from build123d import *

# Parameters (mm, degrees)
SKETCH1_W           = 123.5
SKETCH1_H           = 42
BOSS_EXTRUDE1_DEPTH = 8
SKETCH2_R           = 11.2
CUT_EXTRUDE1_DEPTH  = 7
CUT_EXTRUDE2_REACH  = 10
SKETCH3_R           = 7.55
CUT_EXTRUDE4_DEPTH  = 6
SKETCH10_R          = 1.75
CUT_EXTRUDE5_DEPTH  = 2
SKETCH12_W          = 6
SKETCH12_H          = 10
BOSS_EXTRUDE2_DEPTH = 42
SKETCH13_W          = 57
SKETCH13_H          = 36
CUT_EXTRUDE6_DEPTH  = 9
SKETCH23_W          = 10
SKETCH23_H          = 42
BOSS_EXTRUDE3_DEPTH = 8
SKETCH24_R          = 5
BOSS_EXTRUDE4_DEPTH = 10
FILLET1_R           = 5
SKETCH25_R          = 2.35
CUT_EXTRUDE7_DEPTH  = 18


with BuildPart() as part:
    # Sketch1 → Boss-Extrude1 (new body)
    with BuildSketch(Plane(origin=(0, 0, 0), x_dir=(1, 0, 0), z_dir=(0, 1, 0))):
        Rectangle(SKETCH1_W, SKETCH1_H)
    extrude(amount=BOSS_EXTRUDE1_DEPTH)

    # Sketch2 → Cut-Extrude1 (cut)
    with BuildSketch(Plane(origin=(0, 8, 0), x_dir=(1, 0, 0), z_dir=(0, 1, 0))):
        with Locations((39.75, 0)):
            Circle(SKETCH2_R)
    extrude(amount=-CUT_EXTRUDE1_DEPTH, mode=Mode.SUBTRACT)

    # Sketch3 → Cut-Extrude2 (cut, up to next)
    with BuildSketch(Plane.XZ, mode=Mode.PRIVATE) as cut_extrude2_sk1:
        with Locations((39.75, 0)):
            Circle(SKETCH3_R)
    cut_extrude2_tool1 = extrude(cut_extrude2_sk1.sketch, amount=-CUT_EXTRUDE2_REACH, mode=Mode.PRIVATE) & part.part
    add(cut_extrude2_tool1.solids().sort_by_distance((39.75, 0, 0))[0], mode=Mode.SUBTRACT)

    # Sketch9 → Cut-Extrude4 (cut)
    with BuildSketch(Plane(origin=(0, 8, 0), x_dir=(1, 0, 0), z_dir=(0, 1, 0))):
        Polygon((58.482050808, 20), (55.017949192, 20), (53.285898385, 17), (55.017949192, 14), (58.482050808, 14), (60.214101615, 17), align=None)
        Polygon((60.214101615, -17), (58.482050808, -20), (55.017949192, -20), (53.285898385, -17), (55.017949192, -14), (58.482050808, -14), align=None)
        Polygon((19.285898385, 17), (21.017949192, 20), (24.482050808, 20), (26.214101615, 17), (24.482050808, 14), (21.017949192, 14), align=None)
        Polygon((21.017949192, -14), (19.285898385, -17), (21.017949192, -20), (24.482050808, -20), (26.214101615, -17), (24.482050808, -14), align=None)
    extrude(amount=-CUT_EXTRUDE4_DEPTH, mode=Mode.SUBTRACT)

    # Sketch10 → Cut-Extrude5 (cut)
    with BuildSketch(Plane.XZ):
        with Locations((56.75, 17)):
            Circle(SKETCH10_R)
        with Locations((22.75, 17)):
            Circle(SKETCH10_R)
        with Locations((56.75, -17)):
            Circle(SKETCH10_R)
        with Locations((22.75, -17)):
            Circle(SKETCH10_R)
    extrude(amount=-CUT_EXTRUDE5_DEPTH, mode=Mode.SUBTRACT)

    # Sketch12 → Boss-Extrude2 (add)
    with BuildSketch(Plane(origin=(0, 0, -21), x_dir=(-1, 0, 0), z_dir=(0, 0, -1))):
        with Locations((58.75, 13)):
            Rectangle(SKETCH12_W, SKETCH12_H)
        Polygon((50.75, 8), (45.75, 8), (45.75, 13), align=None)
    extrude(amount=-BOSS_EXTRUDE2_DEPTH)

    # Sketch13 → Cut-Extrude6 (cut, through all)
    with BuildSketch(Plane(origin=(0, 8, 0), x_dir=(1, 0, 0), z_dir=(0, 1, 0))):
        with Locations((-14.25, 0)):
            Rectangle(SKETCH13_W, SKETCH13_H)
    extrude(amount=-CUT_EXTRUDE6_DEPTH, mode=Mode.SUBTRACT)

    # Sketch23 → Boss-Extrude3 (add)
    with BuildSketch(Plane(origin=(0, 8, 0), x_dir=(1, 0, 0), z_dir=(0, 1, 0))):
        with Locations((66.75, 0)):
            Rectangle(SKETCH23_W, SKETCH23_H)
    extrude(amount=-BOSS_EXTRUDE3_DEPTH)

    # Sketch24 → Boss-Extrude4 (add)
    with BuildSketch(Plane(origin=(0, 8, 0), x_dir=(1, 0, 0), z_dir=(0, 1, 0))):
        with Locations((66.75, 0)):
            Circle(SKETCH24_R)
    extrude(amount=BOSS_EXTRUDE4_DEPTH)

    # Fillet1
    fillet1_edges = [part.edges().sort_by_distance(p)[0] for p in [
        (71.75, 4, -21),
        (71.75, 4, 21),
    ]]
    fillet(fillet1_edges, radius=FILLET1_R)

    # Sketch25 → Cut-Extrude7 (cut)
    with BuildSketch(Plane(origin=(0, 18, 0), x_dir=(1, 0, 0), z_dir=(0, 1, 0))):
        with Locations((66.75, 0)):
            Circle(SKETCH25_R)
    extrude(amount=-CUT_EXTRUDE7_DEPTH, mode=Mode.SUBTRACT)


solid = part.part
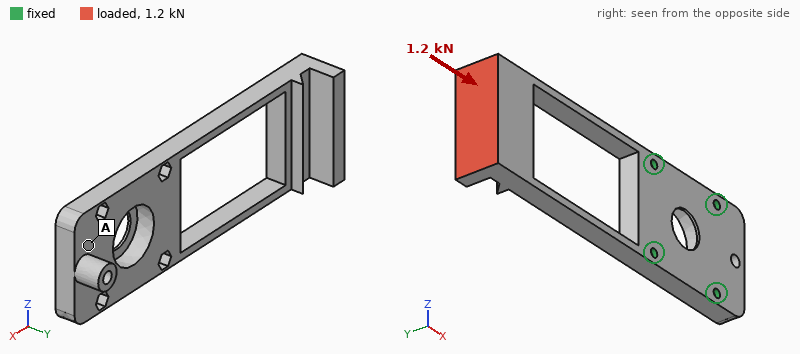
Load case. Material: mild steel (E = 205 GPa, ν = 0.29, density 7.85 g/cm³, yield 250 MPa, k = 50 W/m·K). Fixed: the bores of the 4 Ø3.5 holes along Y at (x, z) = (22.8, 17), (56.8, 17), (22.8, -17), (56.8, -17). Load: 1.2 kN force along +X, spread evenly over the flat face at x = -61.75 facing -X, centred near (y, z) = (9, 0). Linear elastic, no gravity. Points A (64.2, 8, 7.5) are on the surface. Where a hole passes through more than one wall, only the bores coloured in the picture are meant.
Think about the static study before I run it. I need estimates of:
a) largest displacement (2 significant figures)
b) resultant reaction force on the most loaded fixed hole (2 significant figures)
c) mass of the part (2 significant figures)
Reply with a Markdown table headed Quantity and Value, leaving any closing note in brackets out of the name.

| Quantity | Value |
|---|---|
| largest displacement | 0.42 mm |
| resultant reaction force on the most loaded fixed hole | 390 N |
| mass of the part | 220 g |
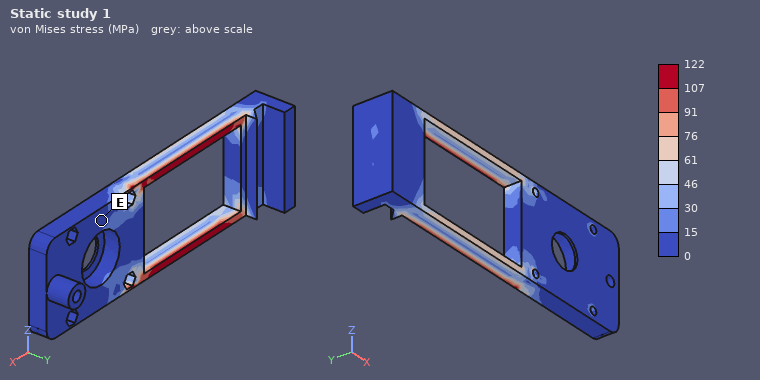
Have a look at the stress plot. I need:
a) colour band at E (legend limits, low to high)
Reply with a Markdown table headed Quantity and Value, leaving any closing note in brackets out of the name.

| Quantity | Value |
|---|---|
| colour band at E | 0 to 15 MPa |
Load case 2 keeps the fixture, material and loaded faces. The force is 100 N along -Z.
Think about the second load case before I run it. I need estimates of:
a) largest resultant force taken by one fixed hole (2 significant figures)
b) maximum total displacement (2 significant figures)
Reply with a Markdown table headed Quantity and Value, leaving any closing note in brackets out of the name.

| Quantity | Value |
|---|---|
| largest resultant force taken by one fixed hole | 200 N |
| maximum total displacement | 0.26 mm |
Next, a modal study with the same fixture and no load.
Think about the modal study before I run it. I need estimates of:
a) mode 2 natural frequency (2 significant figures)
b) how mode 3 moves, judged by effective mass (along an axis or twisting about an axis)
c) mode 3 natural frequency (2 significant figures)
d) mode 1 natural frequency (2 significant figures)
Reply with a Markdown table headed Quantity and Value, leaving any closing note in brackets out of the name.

| Quantity | Value |
|---|---|
| mode 2 natural frequency | 350 Hz |
| how mode 3 moves, judged by effective mass | twisting about X |
| mode 3 natural frequency | 1200 Hz |
| mode 1 natural frequency | 340 Hz |
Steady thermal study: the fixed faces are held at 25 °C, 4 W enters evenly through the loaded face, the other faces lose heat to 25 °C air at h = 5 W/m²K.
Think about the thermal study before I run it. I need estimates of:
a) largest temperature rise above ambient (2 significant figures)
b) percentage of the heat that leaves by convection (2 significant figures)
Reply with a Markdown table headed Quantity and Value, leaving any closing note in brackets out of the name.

| Quantity | Value |
|---|---|
| largest temperature rise above ambient | 75 K |
| percentage of the heat that leaves by convection | 40 % |
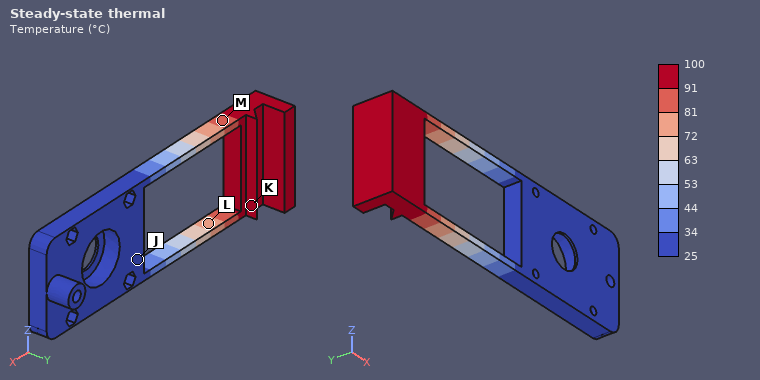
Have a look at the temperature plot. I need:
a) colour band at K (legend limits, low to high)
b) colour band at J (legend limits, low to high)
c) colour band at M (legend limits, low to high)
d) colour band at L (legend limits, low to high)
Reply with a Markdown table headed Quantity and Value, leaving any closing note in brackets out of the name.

| Quantity | Value |
|---|---|
| colour band at K | 91 to 100 °C |
| colour band at J | 25 to 34 °C |
| colour band at M | 81 to 91 °C |
| colour band at L | 72 to 81 °C |
